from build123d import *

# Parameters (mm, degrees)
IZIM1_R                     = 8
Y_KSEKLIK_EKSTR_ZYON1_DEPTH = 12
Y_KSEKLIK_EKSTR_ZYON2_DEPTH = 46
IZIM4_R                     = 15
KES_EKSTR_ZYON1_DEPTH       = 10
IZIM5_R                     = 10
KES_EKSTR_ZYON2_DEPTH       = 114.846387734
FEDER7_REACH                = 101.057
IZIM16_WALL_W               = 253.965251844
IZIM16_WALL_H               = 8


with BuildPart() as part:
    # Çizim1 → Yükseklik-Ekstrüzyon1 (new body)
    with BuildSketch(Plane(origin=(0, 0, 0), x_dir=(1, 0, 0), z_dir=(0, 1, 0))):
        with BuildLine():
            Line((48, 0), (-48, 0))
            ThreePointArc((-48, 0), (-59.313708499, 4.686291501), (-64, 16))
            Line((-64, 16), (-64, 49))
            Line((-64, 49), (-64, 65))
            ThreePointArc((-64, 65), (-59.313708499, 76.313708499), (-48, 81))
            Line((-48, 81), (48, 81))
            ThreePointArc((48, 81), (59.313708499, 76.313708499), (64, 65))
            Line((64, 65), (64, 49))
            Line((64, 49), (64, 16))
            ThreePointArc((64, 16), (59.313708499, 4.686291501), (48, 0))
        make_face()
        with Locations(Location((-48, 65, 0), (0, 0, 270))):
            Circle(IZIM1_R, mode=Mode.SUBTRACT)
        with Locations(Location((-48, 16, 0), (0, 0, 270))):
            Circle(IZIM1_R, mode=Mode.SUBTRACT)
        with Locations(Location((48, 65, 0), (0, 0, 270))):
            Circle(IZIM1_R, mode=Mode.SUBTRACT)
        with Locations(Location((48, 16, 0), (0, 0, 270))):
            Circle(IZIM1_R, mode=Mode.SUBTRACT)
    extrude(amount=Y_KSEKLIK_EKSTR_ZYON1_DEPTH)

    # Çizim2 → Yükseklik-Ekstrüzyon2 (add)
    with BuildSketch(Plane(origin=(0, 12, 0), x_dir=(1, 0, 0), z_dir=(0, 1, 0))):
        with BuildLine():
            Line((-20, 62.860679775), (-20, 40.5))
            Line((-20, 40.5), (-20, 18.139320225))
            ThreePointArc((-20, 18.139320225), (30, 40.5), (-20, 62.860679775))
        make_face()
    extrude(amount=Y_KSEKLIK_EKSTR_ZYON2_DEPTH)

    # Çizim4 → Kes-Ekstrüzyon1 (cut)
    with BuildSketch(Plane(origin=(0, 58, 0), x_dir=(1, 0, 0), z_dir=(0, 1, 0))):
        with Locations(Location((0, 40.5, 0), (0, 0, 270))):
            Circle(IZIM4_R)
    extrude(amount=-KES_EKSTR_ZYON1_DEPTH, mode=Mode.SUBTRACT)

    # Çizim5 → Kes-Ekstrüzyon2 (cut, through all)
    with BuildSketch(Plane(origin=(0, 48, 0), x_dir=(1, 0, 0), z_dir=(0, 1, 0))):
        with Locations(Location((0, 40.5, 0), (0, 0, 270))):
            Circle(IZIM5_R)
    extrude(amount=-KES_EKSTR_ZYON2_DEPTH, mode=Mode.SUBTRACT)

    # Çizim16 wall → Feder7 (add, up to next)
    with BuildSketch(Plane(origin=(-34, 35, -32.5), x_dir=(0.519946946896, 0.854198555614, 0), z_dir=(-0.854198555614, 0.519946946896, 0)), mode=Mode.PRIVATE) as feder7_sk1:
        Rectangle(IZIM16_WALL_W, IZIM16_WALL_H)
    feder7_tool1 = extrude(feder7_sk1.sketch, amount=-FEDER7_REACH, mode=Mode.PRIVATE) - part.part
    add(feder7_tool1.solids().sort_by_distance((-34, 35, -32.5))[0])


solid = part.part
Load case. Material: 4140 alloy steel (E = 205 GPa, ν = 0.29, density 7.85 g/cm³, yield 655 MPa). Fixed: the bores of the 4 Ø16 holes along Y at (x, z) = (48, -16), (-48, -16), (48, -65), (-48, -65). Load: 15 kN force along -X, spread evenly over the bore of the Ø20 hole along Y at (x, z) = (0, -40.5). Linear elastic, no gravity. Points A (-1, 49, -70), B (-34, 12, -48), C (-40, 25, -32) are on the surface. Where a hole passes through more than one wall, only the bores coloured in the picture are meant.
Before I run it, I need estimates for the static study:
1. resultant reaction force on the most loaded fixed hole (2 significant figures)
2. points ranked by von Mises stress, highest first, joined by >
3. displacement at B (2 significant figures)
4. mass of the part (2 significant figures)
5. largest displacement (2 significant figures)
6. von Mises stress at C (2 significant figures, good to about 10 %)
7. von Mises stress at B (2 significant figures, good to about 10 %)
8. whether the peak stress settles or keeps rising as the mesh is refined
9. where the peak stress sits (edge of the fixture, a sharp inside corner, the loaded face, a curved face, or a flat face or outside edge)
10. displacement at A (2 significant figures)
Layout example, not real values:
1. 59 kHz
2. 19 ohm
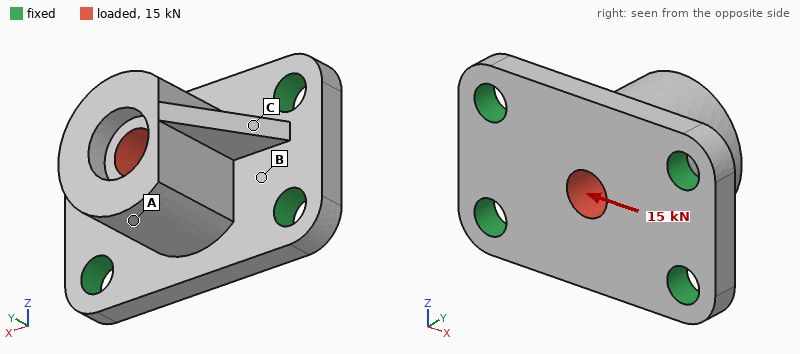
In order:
1. 4.8 kN
2. C > B > A
3. 1.3 µm
4. 1.7 kg
5. 8.4 µm
6. 20 MPa
7. 11 MPa
8. keeps rising
9. edge of the fixture
10. 6.6 µm
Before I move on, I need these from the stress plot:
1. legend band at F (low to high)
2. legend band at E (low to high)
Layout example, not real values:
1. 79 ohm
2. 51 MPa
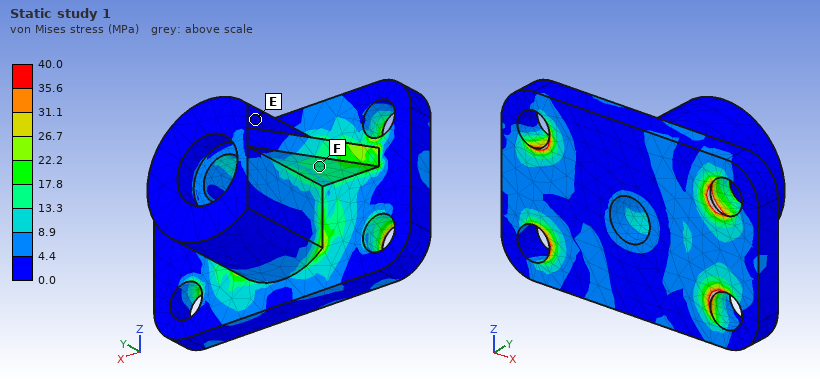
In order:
1. 13.3 to 17.8 MPa
2. 0.0 to 4.4 MPa
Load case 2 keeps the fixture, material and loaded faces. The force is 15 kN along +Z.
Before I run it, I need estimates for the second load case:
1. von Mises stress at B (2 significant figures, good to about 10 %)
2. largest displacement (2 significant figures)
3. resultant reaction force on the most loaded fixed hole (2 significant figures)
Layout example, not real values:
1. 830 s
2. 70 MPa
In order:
1. 30 MPa
2. 23 µm
3. 5.6 kN
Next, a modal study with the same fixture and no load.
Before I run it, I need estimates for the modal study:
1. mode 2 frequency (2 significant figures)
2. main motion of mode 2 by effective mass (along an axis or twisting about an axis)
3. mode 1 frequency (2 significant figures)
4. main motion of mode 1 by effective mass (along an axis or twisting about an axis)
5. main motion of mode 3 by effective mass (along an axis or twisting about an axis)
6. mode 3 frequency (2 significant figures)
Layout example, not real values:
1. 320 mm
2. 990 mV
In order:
1. 6100 Hz
2. along Y
3. 4100 Hz
4. along Z
5. along X
6. 7100 Hz
